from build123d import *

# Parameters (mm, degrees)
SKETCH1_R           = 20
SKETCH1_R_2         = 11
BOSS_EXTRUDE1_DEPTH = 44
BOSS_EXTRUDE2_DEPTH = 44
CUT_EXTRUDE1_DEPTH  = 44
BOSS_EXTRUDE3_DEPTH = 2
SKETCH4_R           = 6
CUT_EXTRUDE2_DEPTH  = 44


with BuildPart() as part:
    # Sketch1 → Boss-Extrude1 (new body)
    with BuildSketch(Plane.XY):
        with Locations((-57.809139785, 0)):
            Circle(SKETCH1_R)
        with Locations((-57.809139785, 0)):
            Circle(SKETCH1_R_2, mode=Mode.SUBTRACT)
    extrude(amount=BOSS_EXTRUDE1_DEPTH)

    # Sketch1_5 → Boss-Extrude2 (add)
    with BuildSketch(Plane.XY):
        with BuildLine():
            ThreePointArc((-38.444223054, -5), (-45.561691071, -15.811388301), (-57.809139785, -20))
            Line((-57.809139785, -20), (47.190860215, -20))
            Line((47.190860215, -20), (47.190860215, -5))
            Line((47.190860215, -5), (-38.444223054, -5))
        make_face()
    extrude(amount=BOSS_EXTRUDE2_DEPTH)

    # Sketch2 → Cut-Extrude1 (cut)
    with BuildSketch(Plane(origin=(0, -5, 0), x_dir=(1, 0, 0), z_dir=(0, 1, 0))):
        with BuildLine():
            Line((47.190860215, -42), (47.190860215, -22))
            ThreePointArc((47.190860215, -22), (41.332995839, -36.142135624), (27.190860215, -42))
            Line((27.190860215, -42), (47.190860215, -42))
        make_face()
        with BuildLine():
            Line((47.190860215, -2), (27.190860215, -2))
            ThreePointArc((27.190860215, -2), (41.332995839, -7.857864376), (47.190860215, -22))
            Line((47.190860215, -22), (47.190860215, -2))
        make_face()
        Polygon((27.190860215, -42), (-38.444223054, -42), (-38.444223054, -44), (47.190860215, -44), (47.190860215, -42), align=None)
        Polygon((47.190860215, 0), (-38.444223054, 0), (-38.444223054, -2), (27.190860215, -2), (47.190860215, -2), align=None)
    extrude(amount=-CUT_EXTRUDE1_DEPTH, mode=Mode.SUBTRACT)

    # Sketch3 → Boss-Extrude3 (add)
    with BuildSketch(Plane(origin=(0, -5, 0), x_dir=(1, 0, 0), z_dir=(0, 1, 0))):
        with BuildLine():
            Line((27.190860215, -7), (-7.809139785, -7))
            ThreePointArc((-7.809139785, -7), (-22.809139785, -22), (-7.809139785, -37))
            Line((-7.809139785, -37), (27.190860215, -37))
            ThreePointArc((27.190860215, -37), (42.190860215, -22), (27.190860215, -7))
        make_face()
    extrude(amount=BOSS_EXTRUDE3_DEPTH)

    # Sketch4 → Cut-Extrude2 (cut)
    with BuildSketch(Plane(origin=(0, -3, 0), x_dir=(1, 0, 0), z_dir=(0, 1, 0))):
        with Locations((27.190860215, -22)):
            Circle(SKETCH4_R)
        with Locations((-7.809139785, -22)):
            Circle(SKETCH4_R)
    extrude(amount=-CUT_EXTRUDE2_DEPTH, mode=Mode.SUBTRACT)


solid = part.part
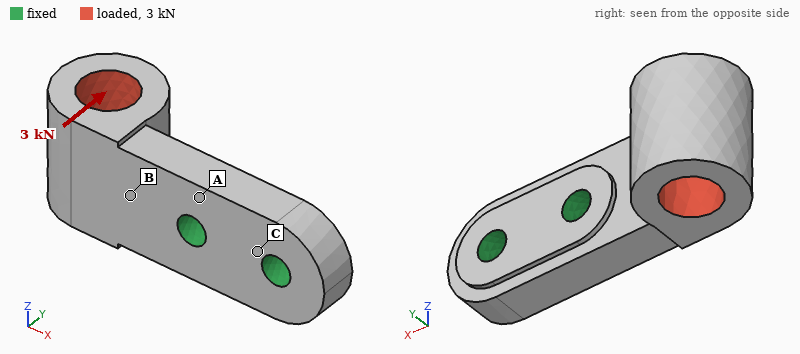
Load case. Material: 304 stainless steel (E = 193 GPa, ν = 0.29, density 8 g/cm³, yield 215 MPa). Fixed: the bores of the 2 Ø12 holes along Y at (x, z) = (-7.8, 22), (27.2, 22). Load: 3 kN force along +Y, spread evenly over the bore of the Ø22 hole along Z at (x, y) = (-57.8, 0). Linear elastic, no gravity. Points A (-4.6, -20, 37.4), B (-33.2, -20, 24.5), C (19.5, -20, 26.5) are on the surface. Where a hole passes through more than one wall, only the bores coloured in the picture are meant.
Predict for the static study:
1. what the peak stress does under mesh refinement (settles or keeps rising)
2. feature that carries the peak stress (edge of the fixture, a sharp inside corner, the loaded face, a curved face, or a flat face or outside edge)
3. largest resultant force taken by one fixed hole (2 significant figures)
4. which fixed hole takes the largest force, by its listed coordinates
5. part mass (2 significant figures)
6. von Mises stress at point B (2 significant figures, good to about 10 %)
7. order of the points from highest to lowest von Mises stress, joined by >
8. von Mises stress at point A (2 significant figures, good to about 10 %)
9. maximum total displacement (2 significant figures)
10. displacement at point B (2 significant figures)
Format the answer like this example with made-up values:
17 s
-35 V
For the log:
keeps rising
edge of the fixture
3.7 kN
(-7.8, 22)
720 g
45 MPa
B > A > C
24 MPa
81 µm
17 µm
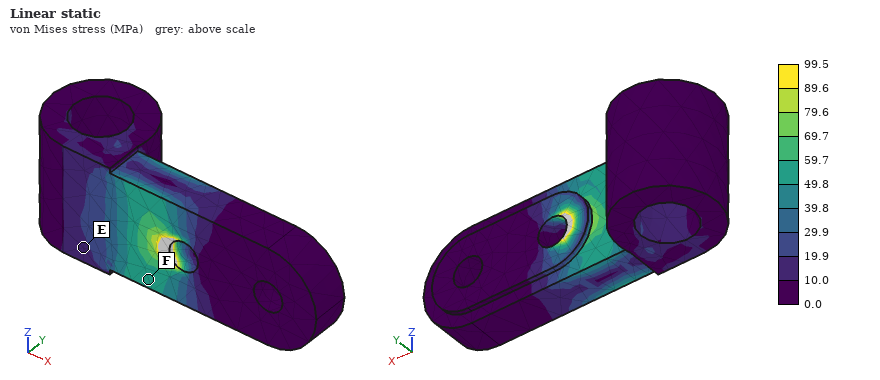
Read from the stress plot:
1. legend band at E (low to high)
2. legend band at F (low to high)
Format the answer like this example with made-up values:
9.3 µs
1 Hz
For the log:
10.0 to 19.9 MPa
49.8 to 59.7 MPa
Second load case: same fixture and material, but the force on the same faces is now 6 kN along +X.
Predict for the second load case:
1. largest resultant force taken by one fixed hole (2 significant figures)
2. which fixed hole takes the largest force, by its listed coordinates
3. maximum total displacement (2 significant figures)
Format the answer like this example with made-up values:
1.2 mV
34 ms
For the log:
5.3 kN
(-7.8, 22)
65 µm
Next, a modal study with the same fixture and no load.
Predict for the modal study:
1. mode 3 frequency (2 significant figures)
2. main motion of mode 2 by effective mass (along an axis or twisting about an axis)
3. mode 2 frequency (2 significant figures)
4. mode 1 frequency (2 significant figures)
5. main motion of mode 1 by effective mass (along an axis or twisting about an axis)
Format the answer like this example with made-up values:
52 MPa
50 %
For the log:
5300 Hz
along Z
3100 Hz
1900 Hz
along Y
